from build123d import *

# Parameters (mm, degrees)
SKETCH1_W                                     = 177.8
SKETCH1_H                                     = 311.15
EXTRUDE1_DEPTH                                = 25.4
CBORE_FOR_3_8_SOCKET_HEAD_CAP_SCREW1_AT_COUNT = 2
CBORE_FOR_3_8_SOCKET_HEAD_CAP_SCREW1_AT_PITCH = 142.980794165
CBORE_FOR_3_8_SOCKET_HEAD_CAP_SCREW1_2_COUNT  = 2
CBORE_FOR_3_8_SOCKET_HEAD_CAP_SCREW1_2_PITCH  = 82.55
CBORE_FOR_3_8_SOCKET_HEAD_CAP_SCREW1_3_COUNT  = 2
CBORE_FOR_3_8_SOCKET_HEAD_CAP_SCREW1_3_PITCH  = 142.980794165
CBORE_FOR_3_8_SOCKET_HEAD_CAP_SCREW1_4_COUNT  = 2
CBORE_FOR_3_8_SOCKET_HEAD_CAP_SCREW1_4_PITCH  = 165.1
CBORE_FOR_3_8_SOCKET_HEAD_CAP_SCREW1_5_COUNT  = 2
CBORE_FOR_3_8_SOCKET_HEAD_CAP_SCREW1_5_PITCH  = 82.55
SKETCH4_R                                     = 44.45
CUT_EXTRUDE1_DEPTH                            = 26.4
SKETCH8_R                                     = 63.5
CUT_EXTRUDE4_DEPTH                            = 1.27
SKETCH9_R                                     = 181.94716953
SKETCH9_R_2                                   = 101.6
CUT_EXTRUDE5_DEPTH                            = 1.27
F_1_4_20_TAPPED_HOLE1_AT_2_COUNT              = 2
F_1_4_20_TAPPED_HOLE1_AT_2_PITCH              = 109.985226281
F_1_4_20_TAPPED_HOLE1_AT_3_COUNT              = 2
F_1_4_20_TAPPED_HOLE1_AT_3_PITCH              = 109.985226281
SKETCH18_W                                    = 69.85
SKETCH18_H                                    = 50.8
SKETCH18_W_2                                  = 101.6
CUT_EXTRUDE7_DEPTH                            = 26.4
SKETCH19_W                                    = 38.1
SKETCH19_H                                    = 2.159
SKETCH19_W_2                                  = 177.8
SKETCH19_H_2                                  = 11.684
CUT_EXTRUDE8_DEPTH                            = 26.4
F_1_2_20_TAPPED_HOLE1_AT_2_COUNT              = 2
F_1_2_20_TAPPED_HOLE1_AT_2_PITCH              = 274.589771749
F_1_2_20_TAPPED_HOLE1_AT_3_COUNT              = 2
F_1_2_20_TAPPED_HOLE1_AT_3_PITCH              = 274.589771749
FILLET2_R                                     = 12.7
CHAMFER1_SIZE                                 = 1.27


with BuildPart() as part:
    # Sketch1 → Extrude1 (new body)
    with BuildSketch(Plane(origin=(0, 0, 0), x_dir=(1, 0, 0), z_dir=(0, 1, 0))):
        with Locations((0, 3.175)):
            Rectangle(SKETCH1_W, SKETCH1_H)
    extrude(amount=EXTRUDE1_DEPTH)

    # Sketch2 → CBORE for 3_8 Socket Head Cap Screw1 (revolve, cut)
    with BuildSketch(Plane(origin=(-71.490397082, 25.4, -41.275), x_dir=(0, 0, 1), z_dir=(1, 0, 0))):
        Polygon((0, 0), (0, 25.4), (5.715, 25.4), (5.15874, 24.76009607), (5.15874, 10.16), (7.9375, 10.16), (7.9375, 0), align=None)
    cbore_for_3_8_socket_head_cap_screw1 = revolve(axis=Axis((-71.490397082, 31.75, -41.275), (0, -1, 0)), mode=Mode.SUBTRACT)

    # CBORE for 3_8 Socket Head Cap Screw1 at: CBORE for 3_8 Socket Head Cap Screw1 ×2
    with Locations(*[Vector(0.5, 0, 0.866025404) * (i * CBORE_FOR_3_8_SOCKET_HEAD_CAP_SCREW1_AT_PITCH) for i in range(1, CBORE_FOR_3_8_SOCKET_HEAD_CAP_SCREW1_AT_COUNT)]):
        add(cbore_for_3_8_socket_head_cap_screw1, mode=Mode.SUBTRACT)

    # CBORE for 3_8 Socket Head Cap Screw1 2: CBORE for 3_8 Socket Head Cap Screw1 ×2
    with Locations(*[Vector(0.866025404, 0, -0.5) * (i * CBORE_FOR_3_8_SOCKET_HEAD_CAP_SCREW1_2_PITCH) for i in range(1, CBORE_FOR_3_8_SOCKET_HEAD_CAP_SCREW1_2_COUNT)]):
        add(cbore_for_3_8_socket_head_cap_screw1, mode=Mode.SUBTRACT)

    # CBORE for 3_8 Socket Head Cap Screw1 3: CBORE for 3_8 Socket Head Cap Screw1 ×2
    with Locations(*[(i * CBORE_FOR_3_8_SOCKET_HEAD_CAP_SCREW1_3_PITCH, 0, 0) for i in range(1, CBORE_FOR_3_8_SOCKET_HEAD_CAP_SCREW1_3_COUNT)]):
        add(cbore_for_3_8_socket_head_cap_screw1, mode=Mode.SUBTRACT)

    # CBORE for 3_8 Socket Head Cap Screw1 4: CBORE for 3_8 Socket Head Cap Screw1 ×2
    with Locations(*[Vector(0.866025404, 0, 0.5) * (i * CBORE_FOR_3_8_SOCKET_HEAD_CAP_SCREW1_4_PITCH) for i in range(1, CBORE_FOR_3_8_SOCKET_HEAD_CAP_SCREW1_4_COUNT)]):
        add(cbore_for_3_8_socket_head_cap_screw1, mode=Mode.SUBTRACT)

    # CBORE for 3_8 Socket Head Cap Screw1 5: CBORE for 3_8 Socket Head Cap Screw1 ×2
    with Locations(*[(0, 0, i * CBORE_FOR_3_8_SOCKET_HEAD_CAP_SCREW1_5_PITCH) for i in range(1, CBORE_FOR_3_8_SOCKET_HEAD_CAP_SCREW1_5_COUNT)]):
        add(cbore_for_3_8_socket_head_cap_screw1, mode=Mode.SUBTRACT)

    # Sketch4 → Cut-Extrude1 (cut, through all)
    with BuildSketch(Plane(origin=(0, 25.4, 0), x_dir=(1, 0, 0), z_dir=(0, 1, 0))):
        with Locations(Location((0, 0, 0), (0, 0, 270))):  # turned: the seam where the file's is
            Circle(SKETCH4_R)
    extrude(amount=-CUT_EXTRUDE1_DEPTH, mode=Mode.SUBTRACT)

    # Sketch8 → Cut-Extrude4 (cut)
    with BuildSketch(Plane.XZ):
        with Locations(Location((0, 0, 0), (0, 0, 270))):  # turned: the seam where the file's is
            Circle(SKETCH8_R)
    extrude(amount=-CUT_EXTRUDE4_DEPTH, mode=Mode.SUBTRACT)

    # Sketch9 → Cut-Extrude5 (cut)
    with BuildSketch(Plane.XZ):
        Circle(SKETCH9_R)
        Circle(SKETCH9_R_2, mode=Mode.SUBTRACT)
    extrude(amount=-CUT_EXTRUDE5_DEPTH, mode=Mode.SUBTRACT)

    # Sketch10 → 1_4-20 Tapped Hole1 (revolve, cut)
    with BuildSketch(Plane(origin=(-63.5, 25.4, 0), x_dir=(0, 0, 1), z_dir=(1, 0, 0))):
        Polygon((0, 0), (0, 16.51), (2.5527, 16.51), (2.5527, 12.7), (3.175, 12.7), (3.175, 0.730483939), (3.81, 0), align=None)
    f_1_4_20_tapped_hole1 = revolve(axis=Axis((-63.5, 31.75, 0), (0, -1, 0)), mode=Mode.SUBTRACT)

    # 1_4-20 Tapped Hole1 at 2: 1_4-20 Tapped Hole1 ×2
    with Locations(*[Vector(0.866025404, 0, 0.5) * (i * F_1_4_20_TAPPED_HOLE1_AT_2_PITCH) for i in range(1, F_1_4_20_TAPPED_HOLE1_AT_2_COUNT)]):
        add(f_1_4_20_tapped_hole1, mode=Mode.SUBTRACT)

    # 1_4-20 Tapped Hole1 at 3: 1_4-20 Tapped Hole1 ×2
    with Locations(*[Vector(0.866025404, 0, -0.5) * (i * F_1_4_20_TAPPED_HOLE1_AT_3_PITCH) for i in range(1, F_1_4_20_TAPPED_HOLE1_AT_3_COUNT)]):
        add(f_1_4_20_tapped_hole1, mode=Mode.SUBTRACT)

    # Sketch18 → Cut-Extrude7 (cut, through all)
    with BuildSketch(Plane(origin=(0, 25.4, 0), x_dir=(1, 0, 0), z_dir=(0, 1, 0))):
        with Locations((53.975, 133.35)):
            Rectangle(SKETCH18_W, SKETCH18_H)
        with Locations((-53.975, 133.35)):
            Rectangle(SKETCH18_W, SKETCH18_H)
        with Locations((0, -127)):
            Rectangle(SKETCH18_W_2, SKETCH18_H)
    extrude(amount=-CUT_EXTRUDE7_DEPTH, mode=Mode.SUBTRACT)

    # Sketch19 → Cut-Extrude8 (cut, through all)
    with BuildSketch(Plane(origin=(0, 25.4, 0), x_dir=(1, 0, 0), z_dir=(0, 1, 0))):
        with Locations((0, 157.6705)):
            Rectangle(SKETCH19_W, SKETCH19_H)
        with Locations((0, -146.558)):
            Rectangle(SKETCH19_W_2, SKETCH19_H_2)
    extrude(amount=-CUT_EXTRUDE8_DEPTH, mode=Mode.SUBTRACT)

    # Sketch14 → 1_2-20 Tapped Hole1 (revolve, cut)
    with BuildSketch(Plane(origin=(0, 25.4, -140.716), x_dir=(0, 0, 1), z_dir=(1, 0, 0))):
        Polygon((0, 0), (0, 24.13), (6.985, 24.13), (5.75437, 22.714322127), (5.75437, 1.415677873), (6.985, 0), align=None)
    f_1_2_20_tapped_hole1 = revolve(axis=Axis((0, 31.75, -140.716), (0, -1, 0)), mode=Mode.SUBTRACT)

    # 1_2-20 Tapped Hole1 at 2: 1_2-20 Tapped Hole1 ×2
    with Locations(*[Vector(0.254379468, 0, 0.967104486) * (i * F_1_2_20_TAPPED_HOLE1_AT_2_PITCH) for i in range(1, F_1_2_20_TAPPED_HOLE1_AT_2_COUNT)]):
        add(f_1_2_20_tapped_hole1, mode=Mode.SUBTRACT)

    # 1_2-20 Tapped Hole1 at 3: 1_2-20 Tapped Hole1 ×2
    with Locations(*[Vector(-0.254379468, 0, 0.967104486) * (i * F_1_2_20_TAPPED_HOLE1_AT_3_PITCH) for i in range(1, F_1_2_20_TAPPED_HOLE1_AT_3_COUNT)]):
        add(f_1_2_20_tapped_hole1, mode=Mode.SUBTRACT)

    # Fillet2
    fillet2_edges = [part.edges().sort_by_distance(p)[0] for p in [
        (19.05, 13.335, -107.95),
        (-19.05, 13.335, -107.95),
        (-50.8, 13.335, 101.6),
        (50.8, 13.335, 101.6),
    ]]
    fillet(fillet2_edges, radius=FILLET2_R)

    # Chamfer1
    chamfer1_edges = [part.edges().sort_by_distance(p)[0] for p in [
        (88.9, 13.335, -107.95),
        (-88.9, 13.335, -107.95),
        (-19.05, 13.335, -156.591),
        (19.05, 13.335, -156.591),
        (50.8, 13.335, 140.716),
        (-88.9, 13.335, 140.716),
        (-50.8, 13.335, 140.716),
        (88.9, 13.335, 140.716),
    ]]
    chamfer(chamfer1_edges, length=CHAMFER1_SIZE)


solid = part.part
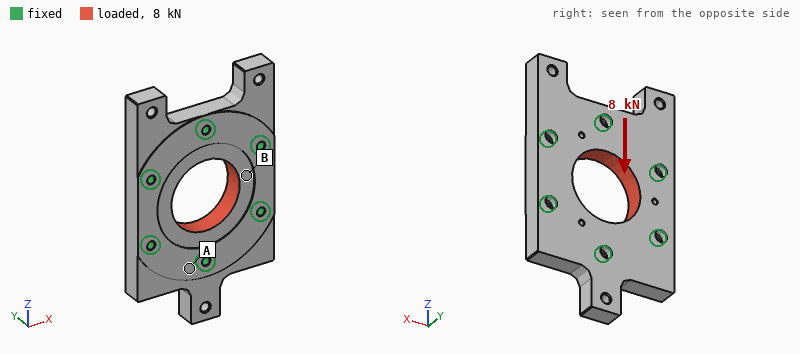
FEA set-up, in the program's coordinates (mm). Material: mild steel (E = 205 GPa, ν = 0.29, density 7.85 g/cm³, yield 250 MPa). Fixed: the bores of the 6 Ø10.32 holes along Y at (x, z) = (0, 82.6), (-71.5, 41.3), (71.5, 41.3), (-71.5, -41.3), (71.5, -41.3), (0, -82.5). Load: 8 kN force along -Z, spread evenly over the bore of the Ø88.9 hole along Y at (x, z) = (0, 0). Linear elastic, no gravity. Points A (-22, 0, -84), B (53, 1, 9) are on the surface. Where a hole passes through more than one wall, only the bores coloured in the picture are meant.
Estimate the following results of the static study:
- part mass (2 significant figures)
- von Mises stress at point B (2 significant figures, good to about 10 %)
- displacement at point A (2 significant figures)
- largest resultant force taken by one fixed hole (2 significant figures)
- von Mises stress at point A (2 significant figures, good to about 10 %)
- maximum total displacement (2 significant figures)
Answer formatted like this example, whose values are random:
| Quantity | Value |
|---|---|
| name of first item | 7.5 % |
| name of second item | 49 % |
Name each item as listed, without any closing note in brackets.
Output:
| Quantity | Value |
|---|---|
| part mass | 6.8 kg |
| von Mises stress at point B | 1.9 MPa |
| displacement at point A | 0.16 µm |
| largest resultant force taken by one fixed hole | 1.7 kN |
| von Mises stress at point A | 0.71 MPa |
| maximum total displacement | 0.73 µm |
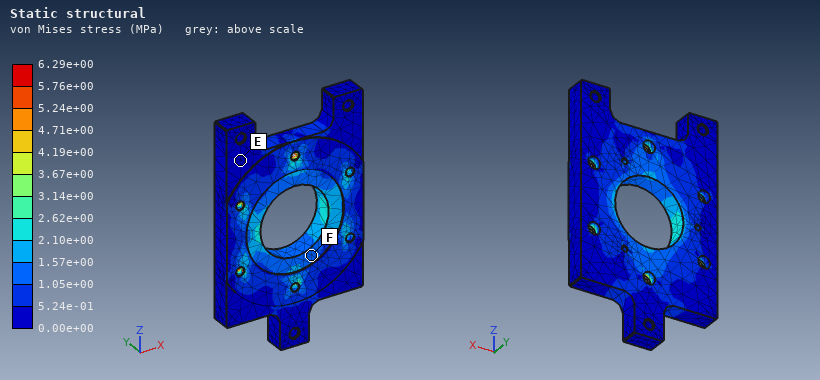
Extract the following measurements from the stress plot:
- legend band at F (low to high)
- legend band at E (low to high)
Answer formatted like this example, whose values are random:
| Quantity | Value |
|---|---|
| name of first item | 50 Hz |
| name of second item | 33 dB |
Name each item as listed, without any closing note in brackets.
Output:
| Quantity | Value |
|---|---|
| legend band at F | 1.05e+00 to 1.57e+00 MPa |
| legend band at E | 0.00e+00 to 5.24e-01 MPa |
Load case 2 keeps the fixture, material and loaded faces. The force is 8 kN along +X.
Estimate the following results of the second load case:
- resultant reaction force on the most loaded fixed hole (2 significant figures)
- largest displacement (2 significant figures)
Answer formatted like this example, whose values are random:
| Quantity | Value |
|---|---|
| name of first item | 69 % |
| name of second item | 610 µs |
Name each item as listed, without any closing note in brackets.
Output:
| Quantity | Value |
|---|---|
| resultant reaction force on the most loaded fixed hole | 1.6 kN |
| largest displacement | 0.74 µm |
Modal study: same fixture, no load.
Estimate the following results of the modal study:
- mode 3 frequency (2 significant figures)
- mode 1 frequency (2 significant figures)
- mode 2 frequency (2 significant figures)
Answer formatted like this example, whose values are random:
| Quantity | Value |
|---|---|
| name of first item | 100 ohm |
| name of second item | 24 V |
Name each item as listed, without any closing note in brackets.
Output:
| Quantity | Value |
|---|---|
| mode 3 frequency | 3400 Hz |
| mode 1 frequency | 2600 Hz |
| mode 2 frequency | 2600 Hz |
